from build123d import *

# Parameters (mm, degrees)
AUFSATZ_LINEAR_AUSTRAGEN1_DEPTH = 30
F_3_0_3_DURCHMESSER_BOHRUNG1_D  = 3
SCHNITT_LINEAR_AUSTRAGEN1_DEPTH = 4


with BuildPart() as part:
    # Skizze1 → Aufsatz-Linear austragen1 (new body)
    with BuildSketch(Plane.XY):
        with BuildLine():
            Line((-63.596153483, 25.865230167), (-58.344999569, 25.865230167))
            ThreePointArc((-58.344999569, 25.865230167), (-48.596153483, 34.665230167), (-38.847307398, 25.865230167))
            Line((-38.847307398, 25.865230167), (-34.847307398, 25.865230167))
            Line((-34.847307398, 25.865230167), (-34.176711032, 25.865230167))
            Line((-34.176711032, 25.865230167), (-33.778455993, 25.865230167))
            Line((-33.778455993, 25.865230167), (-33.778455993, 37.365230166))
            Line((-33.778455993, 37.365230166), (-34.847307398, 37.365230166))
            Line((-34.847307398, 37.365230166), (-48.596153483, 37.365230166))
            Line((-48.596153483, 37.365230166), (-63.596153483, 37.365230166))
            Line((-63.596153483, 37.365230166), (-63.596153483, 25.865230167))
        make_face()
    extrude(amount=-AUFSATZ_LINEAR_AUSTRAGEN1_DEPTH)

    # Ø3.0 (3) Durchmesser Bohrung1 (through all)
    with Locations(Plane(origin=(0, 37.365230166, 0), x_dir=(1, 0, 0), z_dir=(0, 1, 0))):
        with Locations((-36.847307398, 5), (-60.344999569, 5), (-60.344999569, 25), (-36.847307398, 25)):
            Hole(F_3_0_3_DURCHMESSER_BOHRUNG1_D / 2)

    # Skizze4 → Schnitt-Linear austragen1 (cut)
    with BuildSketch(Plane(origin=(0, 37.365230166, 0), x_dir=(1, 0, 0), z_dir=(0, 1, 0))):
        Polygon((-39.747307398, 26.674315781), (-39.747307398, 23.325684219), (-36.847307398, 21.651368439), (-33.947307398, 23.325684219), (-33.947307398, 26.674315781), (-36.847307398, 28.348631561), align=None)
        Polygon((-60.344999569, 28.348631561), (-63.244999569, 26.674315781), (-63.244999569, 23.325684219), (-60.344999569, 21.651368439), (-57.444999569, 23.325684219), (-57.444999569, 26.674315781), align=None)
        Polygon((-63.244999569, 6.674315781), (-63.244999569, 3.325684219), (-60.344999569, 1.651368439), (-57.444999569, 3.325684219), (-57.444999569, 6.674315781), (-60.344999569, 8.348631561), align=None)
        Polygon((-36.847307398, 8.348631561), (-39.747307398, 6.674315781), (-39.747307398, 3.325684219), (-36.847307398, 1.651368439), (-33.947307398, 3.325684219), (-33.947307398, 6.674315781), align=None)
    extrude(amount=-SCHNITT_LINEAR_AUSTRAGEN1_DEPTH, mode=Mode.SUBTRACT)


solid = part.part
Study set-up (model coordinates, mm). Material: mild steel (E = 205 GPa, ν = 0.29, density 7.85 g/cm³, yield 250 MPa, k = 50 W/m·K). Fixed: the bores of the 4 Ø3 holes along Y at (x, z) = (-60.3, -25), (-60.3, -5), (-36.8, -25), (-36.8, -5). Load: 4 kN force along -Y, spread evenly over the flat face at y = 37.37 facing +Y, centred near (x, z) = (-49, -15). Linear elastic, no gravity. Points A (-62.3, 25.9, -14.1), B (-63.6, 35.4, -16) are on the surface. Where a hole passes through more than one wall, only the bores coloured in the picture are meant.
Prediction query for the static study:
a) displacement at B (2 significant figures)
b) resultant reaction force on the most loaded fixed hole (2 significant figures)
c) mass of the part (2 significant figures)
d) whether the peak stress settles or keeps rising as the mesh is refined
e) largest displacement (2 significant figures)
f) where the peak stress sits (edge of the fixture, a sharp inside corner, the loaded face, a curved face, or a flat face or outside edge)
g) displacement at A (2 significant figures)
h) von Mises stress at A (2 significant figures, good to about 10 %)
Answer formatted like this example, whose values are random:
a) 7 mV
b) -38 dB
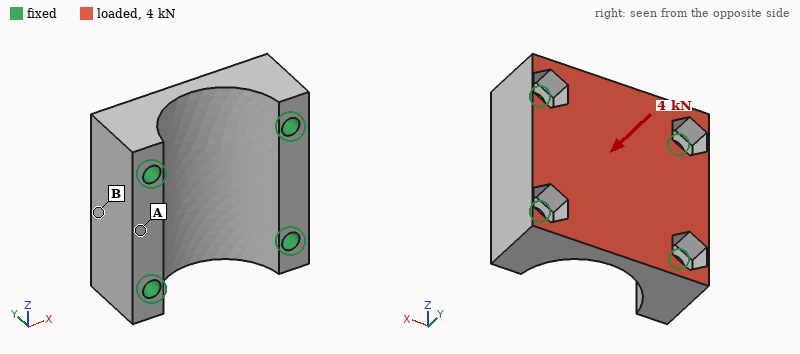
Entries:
a) 0.54 µm
b) 1.2 kN
c) 45 g
d) keeps rising
e) 3.0 µm
f) edge of the fixture
g) 0.99 µm
h) 13 MPa
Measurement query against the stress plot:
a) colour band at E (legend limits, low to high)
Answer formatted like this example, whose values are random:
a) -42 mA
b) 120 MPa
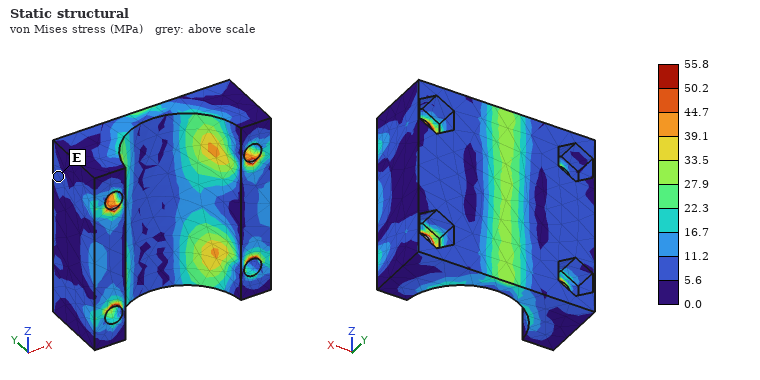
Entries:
a) 5.6 to 11.2 MPa
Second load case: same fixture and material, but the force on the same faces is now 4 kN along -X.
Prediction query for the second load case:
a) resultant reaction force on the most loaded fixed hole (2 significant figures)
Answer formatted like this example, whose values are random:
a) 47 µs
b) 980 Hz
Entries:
a) 1.1 kN
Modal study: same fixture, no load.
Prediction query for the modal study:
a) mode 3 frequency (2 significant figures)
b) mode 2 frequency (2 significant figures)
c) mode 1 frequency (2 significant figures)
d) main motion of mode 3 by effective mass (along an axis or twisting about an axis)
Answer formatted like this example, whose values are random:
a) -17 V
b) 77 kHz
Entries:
a) 52 kHz
b) 45 kHz
c) 44 kHz
d) along Z
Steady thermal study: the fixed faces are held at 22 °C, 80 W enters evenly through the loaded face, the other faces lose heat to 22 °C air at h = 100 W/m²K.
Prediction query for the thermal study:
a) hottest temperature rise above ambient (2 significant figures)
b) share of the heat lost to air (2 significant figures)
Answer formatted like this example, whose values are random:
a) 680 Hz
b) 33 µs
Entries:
a) 50 K
b) 6.2 %
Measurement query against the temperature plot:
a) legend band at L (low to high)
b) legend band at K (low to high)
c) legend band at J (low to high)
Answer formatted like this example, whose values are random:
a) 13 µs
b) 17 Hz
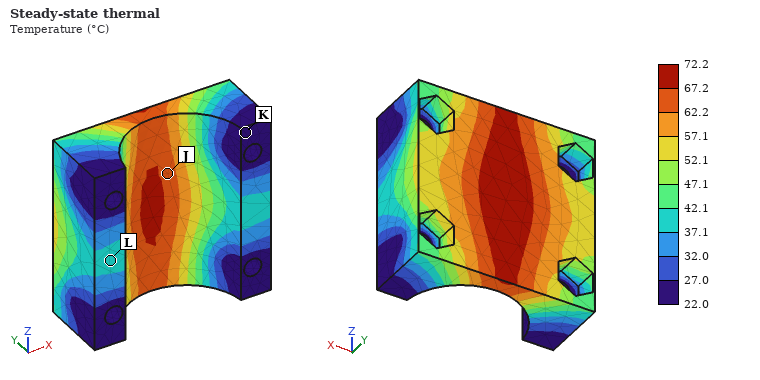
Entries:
a) 37.1 to 42.1 °C
b) 22.0 to 27.0 °C
c) 62.2 to 67.2 °C
